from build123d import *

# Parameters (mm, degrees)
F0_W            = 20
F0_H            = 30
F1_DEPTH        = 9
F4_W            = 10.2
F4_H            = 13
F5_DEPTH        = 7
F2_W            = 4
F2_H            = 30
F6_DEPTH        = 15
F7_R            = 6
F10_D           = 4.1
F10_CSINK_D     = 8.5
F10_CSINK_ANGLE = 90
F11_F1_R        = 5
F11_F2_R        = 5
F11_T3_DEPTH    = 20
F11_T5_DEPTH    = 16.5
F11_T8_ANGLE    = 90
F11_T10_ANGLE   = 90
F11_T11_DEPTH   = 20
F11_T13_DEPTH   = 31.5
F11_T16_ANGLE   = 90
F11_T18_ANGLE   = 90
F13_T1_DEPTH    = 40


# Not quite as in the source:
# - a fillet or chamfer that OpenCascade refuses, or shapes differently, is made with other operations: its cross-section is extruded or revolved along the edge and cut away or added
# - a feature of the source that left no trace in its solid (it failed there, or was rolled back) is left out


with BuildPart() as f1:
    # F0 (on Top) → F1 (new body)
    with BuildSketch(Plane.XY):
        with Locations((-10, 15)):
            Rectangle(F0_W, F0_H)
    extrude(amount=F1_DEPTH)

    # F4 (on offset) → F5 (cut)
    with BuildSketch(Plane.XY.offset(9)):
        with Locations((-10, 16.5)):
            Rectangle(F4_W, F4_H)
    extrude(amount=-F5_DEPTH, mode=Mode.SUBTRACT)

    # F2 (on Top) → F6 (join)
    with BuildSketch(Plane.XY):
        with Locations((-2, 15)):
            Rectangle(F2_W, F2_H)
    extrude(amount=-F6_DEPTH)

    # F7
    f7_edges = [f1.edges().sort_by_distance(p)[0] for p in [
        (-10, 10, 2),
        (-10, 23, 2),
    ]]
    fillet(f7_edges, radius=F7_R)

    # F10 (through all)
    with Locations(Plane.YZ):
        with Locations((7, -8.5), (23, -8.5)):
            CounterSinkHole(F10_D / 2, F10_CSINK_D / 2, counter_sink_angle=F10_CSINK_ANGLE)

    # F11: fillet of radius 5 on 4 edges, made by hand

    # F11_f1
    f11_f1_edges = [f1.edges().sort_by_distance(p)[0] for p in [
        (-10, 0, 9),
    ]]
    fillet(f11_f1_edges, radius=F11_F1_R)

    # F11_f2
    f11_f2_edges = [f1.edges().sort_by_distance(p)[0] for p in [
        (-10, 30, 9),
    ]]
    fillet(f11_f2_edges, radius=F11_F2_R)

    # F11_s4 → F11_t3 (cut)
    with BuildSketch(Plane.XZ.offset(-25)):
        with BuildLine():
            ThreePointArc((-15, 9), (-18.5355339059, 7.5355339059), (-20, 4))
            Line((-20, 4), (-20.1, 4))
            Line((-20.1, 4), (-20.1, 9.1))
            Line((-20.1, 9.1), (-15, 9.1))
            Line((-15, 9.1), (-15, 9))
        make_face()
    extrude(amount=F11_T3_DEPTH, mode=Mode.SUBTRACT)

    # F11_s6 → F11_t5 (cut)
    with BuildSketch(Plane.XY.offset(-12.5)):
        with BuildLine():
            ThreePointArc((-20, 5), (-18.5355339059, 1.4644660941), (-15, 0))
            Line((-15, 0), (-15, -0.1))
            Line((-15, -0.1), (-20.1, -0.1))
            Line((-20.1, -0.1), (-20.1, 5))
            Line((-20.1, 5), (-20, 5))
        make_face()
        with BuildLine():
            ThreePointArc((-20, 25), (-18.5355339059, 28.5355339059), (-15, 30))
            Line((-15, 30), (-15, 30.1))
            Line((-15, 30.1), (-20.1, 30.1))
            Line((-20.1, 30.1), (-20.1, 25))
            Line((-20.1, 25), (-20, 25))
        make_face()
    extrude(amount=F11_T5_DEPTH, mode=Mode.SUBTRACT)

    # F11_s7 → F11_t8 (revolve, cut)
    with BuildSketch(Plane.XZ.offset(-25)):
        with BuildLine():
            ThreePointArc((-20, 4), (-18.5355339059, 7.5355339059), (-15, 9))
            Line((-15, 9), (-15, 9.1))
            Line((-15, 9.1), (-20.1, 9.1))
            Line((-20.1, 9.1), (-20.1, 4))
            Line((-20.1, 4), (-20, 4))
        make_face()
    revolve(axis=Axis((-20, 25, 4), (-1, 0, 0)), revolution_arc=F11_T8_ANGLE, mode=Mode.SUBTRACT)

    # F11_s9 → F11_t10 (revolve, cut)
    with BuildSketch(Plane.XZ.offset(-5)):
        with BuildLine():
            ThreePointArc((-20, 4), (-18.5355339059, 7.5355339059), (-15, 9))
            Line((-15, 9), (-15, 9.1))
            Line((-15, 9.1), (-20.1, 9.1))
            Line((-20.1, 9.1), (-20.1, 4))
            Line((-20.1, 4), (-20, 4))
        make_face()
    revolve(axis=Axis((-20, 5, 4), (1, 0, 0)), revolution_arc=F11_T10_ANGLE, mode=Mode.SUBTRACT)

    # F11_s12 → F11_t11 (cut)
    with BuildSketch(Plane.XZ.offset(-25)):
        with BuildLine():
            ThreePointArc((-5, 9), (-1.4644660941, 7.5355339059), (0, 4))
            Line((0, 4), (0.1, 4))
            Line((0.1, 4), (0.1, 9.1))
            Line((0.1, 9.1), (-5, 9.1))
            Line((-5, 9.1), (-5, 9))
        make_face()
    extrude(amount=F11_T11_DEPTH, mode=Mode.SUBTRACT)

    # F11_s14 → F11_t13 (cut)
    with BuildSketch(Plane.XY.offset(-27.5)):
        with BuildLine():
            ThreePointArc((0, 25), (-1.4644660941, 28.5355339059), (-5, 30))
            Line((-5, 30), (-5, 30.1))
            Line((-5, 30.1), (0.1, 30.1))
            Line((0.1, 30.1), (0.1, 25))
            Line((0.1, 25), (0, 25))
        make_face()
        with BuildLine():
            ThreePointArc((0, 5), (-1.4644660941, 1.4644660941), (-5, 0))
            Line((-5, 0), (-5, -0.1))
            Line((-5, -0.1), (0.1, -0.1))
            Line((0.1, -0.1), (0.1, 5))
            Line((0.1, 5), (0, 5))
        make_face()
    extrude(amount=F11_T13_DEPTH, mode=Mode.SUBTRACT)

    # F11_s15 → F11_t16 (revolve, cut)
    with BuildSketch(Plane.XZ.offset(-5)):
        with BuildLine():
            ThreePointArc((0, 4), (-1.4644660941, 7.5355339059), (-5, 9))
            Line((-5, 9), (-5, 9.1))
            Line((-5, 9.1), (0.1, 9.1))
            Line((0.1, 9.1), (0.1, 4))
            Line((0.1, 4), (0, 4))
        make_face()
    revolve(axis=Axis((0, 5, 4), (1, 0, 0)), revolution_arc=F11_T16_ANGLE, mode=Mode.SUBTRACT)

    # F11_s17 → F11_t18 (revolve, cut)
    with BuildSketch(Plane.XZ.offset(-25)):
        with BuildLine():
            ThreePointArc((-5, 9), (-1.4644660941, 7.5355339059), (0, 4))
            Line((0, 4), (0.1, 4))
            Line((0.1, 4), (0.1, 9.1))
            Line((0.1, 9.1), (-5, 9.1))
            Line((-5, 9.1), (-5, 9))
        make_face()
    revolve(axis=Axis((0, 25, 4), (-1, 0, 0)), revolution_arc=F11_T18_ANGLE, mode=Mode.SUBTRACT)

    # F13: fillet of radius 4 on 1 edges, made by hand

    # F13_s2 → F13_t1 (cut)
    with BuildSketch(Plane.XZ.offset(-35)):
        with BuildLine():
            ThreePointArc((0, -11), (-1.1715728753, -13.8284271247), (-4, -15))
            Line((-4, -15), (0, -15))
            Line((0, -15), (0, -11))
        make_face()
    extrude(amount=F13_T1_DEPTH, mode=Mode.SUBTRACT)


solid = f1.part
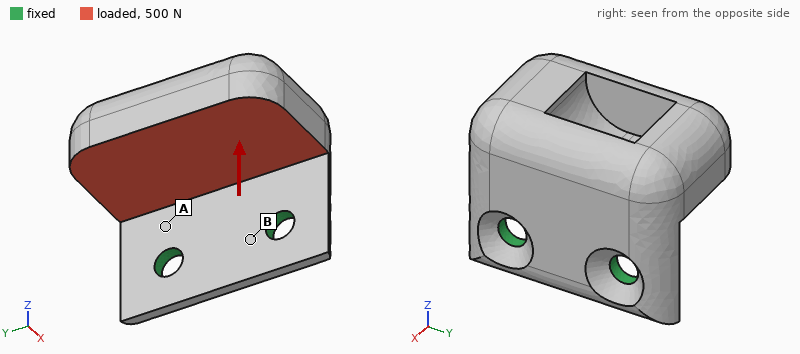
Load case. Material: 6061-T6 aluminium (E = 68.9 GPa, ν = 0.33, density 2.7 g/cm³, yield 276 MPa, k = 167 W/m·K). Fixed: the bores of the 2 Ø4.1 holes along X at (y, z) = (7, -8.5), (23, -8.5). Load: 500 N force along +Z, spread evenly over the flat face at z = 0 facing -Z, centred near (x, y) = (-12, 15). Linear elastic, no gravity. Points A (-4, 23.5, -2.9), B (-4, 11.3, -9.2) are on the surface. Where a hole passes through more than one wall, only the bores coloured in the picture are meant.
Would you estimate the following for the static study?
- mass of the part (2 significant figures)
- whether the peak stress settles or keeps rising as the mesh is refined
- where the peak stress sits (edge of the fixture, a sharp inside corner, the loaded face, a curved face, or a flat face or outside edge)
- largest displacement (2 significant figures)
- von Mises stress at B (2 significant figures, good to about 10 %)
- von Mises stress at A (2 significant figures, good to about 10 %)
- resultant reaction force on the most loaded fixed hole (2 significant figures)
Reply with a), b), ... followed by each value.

a) 14 g
b) keeps rising
c) edge of the fixture
d) 0.14 mm
e) 33 MPa
f) 71 MPa
g) 260 N
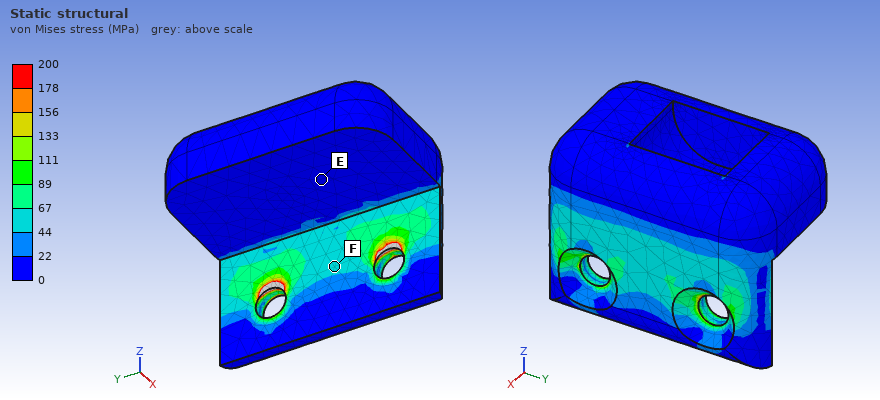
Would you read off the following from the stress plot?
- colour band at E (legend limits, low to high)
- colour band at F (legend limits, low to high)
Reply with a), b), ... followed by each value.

a) 0 to 22 MPa
b) 44 to 67 MPa
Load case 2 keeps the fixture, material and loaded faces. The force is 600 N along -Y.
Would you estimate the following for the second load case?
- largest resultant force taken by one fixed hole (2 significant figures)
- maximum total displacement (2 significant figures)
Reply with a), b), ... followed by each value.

a) 480 N
b) 43 µm
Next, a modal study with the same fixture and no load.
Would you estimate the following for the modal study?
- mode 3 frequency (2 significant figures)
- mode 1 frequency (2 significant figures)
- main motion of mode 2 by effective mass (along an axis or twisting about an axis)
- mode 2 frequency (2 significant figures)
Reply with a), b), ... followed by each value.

a) 12 kHz
b) 3000 Hz
c) along Y
d) 6500 Hz
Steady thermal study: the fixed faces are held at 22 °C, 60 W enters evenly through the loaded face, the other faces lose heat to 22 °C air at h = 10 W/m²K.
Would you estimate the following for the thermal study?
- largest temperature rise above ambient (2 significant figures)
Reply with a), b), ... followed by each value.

a) 58 K
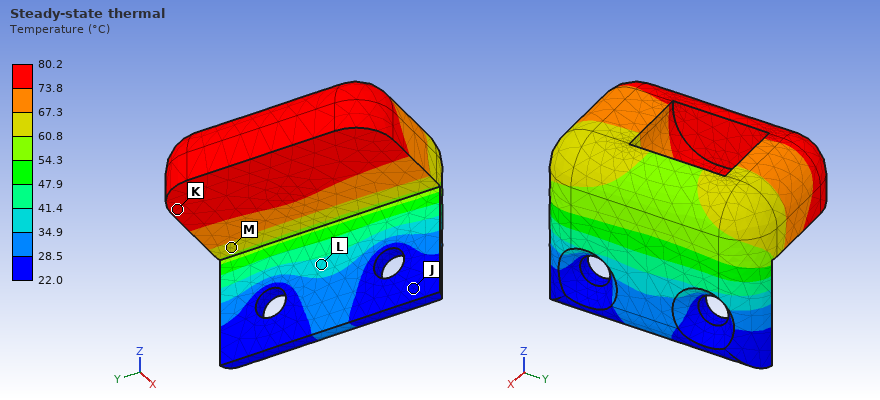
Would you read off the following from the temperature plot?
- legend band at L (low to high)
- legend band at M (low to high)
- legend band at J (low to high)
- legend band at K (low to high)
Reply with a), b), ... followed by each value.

a) 34.9 to 41.4 °C
b) 60.8 to 67.3 °C
c) 22.0 to 28.5 °C
d) 73.8 to 80.2 °C
